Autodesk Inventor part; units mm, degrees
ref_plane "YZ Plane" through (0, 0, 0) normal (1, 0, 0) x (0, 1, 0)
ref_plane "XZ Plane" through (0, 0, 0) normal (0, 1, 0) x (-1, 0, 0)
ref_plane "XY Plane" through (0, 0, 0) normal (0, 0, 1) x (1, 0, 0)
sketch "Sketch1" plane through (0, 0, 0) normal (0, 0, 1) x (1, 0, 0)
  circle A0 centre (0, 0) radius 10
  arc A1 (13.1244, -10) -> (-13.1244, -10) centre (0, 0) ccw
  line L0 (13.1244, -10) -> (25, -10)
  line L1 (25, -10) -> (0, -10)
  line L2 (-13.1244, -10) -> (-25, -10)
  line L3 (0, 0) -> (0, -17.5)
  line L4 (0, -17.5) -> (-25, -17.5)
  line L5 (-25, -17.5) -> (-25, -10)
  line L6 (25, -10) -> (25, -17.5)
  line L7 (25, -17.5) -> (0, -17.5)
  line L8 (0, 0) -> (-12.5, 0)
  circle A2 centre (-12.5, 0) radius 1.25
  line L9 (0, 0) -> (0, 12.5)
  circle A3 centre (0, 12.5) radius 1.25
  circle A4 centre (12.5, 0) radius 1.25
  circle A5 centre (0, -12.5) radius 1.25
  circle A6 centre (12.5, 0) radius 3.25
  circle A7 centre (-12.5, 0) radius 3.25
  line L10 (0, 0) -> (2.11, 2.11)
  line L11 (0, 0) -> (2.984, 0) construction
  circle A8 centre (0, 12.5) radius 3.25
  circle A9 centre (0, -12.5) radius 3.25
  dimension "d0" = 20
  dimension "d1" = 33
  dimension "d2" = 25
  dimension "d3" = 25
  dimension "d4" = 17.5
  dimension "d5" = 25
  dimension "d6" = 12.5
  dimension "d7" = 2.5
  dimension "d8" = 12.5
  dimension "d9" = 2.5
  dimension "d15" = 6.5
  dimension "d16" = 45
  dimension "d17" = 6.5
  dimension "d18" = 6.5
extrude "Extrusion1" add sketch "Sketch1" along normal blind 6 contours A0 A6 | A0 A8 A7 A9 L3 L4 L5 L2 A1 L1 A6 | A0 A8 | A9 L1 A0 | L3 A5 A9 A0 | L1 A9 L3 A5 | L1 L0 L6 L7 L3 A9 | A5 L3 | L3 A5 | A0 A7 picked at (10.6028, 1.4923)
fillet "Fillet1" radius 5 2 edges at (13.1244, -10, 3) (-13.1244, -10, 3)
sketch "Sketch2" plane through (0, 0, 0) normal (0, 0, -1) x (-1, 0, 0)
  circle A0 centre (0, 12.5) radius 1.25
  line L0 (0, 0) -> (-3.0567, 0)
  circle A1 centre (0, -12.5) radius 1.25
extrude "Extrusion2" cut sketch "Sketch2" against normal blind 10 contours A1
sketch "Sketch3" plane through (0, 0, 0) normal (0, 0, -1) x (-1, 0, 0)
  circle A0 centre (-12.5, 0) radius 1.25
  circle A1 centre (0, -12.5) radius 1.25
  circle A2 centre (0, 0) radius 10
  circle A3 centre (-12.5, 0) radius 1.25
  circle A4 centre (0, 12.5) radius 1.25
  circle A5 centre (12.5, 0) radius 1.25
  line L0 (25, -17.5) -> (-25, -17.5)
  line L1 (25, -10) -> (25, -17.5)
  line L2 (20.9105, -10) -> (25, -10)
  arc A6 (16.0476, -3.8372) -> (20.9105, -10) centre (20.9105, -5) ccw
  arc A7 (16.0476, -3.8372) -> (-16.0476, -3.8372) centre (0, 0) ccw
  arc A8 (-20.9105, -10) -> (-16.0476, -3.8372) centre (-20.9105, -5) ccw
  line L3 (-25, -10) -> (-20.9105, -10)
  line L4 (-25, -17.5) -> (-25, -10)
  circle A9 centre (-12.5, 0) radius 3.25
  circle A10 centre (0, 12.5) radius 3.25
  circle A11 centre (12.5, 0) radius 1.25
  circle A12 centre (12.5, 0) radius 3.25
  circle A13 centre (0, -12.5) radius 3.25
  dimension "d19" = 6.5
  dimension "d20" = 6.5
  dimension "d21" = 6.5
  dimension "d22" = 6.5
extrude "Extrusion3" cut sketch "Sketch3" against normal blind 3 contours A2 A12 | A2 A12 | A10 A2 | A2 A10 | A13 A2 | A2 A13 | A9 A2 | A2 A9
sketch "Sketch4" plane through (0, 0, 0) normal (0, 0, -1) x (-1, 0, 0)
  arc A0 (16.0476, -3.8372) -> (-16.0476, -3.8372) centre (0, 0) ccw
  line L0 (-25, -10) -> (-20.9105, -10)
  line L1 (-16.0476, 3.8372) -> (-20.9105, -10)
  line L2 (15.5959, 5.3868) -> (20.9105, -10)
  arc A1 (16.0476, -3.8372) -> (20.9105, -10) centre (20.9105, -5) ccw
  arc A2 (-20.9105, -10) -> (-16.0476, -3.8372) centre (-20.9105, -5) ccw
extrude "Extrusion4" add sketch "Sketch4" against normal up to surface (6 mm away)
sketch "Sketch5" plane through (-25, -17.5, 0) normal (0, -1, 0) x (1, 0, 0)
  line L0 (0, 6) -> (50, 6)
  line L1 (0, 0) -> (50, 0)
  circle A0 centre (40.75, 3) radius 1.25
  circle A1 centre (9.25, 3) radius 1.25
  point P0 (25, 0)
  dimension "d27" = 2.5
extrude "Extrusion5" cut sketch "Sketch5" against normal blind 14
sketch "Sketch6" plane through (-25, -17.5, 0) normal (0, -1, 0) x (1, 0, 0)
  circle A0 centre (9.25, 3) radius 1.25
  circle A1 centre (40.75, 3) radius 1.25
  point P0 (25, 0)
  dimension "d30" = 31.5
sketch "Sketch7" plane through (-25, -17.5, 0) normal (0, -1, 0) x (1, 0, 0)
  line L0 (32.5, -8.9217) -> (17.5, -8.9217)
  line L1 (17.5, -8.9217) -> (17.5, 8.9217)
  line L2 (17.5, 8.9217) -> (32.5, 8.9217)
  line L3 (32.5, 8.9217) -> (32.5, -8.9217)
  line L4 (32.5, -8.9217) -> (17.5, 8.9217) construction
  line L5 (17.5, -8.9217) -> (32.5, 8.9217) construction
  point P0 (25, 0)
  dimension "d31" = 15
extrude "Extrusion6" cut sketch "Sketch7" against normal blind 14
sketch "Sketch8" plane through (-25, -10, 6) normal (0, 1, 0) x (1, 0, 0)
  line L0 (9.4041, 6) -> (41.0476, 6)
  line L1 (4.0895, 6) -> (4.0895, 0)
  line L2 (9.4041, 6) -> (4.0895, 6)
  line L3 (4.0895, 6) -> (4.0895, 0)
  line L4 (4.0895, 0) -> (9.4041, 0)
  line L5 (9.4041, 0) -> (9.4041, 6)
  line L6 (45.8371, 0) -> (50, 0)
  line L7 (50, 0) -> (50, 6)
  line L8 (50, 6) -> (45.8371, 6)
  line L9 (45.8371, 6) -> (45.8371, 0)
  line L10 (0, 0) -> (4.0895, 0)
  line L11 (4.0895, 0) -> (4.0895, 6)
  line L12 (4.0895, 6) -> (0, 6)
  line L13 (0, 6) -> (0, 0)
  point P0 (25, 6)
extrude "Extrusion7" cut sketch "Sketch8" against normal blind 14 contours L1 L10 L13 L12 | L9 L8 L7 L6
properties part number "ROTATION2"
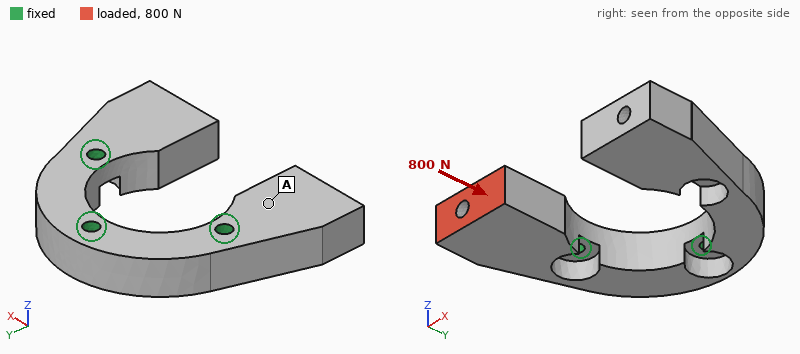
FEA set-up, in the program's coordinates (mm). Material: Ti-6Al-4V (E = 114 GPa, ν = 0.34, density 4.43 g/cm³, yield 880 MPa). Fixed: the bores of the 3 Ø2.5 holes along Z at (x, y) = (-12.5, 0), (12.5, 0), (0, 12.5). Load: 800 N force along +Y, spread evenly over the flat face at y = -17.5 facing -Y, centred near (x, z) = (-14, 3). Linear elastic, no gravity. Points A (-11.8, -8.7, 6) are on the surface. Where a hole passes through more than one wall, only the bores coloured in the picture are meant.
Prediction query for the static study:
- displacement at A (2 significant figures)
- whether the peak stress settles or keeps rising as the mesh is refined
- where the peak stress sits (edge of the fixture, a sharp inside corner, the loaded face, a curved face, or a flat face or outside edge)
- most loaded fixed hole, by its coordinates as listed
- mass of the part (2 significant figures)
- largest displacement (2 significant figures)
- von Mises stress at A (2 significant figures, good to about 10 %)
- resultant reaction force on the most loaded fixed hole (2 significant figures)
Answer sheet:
6.7 µm
keeps rising
edge of the fixture
(-12.5, 0)
16 g
17 µm
15 MPa
770 N
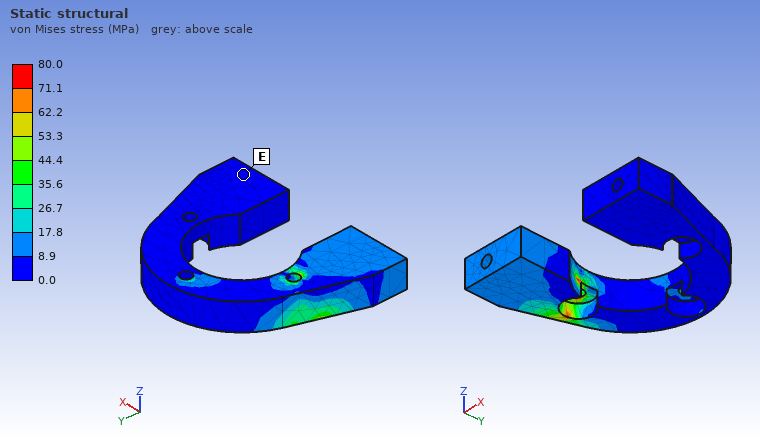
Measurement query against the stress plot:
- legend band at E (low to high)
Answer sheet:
0.0 to 8.9 MPa
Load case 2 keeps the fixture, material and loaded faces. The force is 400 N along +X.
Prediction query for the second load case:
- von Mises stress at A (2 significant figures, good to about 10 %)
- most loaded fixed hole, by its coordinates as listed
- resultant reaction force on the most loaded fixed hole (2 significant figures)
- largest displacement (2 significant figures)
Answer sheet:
26 MPa
(-12.5, 0)
760 N
65 µm
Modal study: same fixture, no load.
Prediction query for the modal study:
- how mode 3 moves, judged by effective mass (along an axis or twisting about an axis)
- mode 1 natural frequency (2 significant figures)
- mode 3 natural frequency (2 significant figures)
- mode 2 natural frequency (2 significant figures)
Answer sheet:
along X
6700 Hz
9700 Hz
6800 Hz
